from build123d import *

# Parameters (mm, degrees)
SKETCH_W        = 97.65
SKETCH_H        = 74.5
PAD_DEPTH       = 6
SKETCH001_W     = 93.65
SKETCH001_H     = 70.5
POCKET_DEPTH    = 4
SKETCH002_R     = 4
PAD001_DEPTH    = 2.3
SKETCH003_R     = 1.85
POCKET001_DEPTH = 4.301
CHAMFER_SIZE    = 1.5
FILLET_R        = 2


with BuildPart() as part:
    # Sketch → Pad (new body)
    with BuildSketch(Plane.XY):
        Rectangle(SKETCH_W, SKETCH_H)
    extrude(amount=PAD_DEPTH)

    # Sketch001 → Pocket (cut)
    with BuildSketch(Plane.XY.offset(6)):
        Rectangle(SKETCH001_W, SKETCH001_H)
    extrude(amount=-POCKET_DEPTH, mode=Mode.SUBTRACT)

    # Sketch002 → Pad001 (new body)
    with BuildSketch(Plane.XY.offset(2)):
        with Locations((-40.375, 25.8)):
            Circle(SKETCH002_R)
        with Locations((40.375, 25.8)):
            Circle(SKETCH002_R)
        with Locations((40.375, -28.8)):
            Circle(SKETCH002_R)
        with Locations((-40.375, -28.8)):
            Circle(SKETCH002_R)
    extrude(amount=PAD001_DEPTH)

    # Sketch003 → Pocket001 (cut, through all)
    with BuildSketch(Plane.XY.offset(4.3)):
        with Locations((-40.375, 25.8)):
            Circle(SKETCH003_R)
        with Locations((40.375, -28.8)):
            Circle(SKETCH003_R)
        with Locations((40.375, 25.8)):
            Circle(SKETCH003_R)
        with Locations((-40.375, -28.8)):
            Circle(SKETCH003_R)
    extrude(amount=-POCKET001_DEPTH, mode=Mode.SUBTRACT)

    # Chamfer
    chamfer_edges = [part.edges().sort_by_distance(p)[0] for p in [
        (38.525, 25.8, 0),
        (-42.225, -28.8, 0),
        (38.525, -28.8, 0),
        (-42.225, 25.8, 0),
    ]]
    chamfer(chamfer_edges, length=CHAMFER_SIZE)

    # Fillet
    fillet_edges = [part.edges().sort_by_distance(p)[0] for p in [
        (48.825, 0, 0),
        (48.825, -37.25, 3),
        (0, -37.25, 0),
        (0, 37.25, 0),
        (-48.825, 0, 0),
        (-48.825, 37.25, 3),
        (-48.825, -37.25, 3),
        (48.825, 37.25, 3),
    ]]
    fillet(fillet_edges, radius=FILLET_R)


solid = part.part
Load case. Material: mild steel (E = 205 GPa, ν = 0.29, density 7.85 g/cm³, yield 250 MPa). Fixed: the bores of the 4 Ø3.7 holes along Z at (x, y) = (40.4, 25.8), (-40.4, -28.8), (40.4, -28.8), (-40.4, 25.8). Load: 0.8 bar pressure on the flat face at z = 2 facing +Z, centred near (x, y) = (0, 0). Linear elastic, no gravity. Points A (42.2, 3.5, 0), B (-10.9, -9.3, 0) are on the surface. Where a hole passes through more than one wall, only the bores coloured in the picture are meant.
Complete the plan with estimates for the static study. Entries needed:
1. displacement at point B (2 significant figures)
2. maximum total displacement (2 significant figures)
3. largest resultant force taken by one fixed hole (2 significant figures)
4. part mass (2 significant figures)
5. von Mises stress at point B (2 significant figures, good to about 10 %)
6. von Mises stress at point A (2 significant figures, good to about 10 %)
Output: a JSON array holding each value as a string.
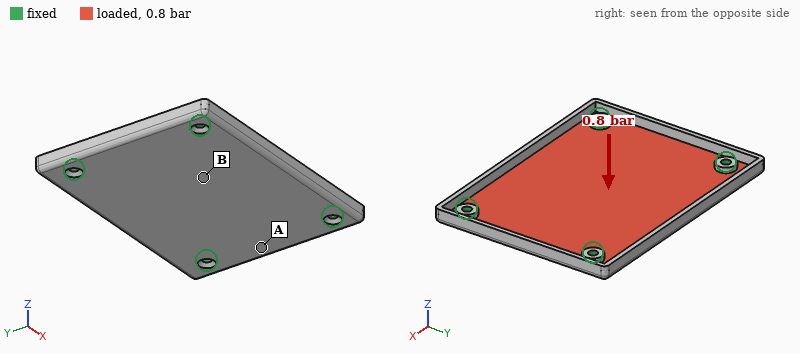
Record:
["54 µm", "63 µm", "170 N", "130 g", "23 MPa", "13 MPa"]
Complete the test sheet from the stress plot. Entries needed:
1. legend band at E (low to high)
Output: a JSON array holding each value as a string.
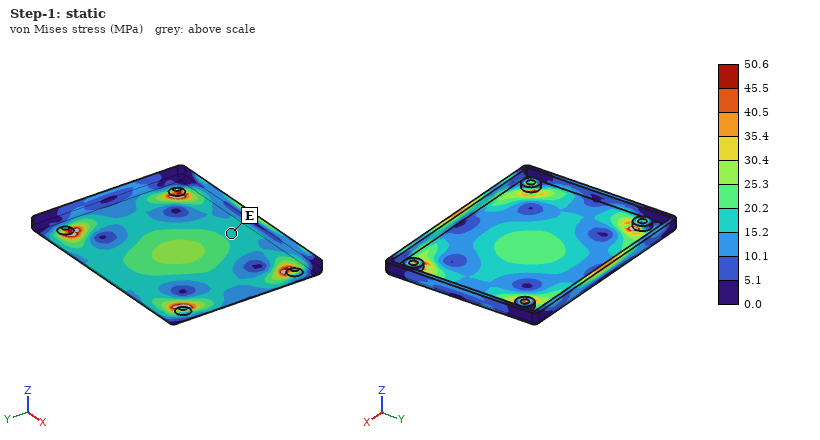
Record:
["15.2 to 20.2 MPa"]
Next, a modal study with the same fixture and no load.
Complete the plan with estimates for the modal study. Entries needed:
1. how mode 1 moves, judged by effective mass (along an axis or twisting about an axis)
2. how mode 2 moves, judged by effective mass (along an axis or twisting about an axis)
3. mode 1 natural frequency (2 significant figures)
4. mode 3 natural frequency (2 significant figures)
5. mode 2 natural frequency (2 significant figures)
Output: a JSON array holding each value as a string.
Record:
["along Z", "twisting about X", "1800 Hz", "3500 Hz", "2700 Hz"]
